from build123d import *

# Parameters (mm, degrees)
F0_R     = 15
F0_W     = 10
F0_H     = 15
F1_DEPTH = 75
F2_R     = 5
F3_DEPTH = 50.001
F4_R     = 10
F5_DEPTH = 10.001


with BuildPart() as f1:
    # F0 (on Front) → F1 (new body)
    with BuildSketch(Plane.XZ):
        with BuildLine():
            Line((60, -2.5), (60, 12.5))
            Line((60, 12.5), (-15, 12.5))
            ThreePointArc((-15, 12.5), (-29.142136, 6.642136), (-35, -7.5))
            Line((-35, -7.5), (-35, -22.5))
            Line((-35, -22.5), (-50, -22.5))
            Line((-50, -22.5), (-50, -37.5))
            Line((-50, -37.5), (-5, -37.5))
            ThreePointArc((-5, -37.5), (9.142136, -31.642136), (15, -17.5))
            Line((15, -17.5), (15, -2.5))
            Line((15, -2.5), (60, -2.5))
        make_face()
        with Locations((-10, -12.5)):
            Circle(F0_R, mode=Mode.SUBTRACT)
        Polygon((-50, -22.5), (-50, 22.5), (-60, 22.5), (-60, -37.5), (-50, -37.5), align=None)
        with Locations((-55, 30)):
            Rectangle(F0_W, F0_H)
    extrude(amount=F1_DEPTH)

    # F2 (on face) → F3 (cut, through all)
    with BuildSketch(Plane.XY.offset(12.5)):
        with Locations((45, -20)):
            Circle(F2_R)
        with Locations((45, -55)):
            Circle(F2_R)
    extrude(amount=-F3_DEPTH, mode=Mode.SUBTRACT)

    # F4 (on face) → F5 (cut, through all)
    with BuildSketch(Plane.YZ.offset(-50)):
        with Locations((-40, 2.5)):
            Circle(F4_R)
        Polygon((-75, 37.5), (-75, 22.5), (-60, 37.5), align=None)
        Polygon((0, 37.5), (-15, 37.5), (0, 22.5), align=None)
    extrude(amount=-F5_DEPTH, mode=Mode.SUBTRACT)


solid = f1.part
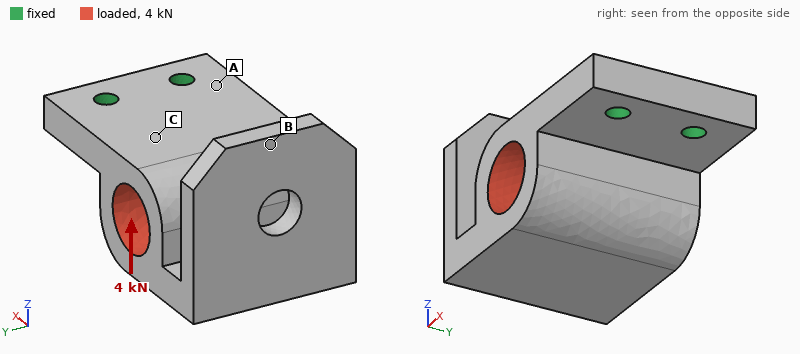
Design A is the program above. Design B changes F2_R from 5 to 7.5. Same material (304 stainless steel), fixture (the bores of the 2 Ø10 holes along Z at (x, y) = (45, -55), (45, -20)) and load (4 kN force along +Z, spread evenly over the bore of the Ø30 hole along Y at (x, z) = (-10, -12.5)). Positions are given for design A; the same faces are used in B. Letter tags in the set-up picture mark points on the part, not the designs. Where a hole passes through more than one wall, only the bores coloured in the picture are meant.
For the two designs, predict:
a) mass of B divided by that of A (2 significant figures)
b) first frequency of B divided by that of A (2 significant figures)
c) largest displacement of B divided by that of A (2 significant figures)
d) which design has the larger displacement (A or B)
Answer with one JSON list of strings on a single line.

["0.99", "1.1", "0.85", "A"]
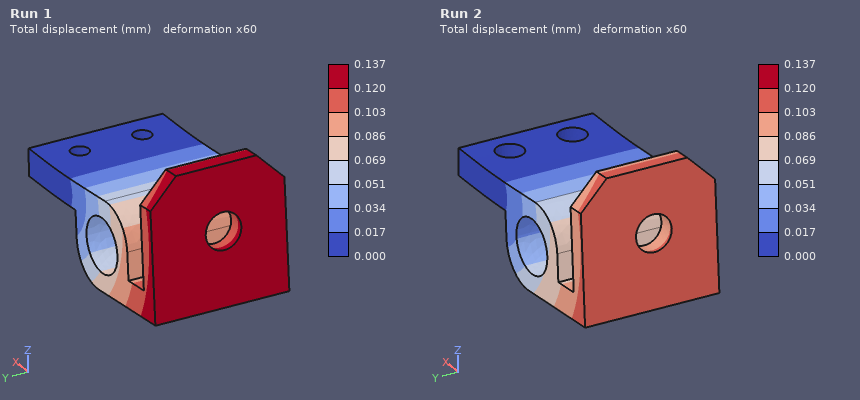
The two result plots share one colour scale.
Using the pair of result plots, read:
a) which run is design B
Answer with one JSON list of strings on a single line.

["Run 2"]
